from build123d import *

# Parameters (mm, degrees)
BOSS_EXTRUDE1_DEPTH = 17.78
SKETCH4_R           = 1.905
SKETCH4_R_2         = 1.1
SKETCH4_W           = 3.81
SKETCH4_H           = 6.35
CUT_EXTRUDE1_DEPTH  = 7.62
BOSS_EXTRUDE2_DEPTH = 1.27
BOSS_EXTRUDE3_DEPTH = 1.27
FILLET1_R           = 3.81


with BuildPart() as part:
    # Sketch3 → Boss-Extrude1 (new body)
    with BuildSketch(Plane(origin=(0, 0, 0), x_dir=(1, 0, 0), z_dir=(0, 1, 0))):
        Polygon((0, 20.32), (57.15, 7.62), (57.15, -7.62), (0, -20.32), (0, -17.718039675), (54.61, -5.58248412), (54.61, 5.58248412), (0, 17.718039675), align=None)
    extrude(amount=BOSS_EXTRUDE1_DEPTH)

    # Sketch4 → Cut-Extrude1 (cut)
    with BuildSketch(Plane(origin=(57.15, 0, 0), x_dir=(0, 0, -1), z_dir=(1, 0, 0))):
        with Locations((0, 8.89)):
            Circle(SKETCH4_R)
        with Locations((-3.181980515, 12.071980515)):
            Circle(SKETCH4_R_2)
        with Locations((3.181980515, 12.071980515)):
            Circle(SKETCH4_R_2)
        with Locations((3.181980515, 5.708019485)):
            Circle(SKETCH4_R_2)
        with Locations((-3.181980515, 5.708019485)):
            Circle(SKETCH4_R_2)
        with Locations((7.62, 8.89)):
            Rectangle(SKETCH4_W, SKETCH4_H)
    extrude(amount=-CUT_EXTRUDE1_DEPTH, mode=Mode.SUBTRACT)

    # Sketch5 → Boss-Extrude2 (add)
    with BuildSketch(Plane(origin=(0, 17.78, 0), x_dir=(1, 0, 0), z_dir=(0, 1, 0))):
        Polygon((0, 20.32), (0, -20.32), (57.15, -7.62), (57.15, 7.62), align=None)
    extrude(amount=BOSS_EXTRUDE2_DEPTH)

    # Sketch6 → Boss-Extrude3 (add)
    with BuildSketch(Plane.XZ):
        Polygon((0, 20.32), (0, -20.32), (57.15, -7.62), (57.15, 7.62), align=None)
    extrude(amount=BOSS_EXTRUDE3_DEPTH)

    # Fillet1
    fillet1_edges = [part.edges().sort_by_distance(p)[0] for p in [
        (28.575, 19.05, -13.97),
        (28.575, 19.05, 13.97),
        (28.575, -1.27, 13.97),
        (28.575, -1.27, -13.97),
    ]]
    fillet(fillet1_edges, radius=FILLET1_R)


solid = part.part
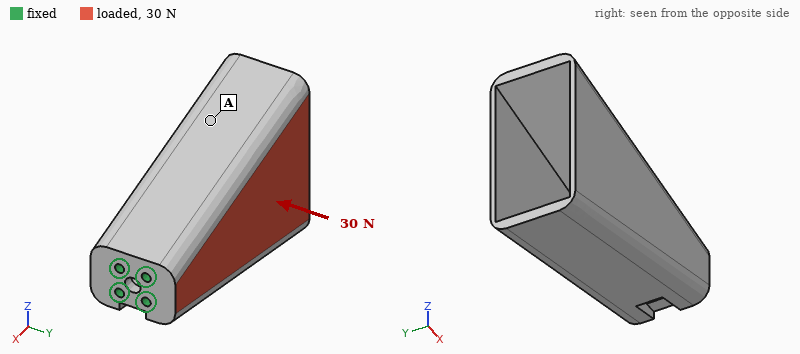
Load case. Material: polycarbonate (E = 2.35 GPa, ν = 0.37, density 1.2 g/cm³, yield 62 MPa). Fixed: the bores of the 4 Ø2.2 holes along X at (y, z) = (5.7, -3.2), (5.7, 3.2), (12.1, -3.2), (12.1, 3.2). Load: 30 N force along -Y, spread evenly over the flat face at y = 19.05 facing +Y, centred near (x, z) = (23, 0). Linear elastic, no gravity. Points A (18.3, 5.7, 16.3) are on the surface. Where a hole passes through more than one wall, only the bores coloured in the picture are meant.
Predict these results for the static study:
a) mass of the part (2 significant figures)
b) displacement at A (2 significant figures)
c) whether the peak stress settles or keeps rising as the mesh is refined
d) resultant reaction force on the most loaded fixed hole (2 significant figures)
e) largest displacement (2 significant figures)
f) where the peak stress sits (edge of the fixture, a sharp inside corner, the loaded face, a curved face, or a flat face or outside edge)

11 g
0.25 mm
keeps rising
54 N
0.70 mm
edge of the fixture
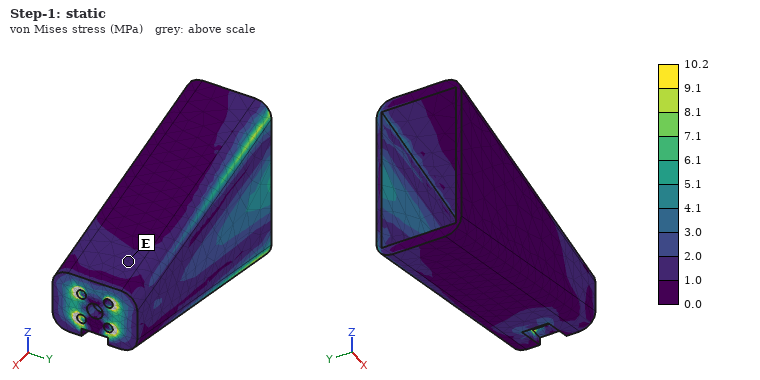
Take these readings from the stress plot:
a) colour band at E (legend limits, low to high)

1.0 to 2.0 MPa
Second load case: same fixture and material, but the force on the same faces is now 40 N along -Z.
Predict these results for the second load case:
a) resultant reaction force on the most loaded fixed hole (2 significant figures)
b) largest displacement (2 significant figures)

83 N
0.74 mm
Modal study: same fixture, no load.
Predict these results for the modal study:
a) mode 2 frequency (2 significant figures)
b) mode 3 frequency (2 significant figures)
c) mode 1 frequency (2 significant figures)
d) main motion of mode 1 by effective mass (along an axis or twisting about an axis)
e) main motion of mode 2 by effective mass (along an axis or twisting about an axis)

540 Hz
1000 Hz
510 Hz
along Z
along Y
